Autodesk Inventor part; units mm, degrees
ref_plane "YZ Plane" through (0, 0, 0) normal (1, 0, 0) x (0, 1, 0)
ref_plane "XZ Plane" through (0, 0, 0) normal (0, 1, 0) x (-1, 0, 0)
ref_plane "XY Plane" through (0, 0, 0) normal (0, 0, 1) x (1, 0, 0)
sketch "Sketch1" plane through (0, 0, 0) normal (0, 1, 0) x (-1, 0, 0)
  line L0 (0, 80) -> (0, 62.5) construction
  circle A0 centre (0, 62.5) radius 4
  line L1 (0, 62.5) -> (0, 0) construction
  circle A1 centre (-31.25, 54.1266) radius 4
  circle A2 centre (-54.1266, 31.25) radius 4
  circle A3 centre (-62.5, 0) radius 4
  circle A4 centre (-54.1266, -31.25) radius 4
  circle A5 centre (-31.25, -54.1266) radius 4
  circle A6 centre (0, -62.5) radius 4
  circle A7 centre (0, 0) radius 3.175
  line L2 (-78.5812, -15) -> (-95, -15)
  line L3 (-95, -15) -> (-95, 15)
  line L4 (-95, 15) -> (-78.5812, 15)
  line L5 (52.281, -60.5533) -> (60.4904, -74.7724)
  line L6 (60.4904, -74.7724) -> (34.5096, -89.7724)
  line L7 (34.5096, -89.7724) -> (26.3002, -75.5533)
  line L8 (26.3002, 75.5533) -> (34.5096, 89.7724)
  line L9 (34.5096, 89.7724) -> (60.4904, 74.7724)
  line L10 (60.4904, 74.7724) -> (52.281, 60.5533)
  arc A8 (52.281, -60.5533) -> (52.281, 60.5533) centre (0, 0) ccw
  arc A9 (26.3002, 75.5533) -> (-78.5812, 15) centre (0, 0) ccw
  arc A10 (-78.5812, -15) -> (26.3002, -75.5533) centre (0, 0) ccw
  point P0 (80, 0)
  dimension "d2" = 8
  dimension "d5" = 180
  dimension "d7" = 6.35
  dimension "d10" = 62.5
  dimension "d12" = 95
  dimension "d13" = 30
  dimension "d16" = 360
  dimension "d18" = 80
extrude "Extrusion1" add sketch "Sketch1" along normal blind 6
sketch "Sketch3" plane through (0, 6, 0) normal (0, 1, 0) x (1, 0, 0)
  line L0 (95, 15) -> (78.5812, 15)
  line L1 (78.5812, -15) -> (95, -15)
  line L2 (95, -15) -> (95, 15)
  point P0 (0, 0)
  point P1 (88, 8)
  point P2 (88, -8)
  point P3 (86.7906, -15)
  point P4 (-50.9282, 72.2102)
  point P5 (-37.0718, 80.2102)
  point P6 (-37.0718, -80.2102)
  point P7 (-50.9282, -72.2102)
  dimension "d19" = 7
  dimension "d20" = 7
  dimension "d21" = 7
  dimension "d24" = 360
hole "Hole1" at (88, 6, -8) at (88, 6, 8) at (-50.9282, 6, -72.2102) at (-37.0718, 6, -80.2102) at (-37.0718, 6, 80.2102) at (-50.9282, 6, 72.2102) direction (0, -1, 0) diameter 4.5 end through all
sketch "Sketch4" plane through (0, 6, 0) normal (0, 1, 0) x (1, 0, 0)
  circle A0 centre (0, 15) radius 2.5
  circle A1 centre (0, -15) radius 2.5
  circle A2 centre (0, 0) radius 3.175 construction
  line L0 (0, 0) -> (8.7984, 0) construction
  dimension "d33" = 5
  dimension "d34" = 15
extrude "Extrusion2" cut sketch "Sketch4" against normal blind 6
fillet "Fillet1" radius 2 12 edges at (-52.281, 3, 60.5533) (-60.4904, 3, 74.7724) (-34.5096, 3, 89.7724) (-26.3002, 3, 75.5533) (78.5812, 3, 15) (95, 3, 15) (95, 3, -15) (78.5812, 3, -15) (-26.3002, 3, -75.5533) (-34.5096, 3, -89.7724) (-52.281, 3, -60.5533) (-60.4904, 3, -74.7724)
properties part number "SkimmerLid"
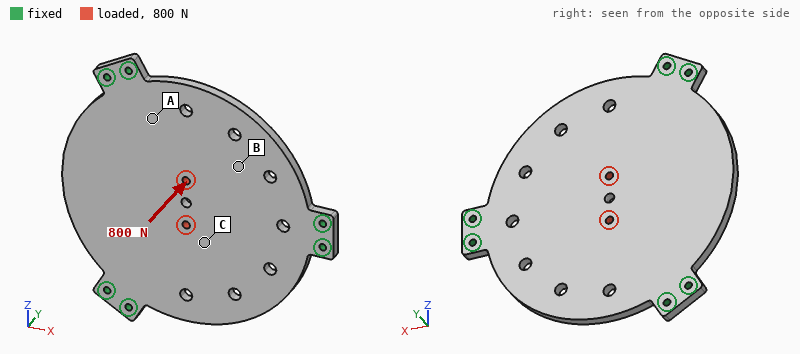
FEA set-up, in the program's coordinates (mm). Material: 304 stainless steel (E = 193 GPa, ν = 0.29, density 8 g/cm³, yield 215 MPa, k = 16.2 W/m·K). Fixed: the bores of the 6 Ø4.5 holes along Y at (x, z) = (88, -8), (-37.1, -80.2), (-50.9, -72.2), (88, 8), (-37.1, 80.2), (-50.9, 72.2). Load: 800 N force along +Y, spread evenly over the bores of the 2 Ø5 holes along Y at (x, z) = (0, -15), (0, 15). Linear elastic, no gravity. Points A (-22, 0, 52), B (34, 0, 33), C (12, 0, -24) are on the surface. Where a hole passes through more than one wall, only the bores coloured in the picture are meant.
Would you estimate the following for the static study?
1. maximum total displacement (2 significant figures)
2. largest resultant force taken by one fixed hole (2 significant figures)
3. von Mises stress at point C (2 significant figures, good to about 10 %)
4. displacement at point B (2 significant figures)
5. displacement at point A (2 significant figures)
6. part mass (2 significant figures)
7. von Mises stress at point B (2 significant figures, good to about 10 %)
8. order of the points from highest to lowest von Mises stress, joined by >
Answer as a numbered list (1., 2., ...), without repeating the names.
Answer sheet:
1. 57 µm
2. 150 N
3. 19 MPa
4. 33 µm
5. 21 µm
6. 1.0 kg
7. 12 MPa
8. C > B > A
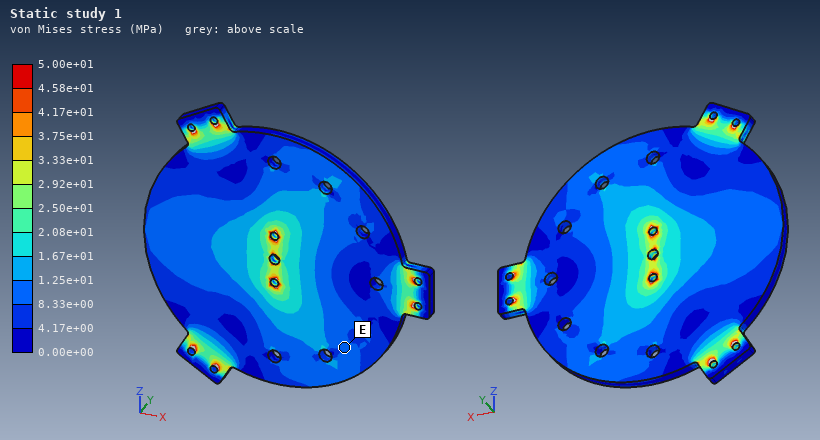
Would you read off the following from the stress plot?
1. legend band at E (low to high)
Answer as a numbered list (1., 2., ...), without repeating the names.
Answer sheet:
1. 8.33e+00 to 1.25e+01 MPa
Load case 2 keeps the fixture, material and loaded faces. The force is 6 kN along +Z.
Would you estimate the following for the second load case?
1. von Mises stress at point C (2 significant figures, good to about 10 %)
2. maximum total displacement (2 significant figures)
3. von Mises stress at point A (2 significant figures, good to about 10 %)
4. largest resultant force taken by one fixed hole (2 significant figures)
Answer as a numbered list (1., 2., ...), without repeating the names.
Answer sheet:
1. 6.4 MPa
2. 6.3 µm
3. 11 MPa
4. 1.5 kN
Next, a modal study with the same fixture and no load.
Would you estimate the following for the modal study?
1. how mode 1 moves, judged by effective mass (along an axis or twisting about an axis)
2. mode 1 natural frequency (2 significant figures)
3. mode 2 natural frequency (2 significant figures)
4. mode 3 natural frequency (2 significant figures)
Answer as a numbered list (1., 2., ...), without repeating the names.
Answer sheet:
1. along Y
2. 1000 Hz
3. 1200 Hz
4. 1200 Hz
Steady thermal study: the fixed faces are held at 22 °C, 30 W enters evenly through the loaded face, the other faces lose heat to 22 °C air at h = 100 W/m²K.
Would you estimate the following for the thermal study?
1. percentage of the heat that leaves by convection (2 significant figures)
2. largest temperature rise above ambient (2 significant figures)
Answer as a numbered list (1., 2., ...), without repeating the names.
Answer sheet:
1. 98 %
2. 67 K
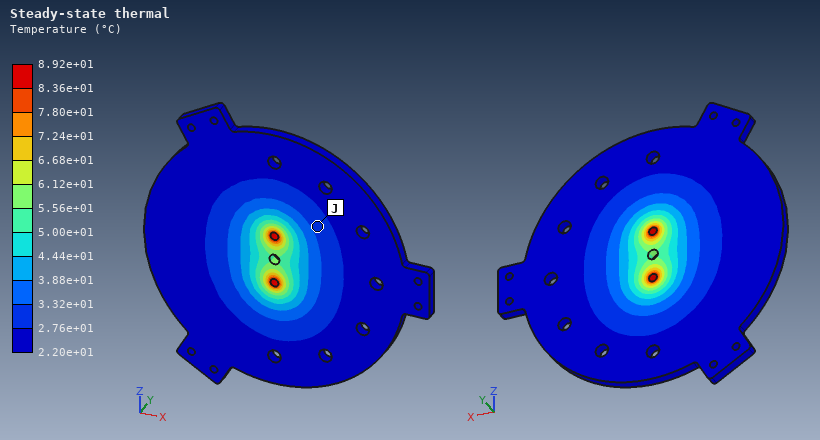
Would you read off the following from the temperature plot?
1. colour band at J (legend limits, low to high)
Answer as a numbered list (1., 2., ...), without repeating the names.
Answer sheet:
1. 2.76e+01 to 3.32e+01 °C
